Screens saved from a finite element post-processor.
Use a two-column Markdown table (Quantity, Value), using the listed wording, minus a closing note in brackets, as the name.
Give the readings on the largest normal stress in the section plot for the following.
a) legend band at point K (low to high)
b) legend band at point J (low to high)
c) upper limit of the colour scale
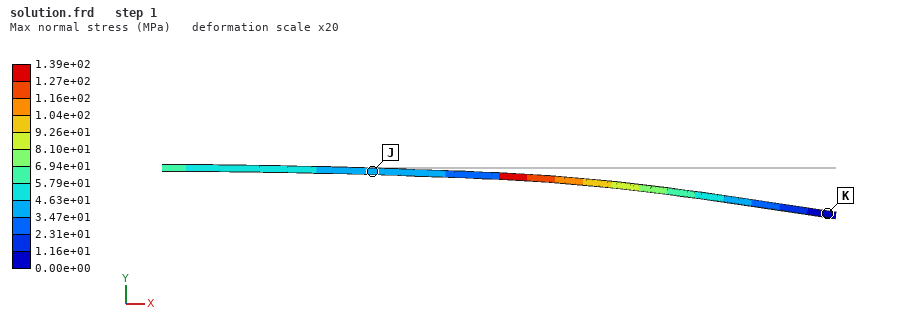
| Quantity | Value |
|---|---|
| legend band at point K | 0.00e+00 to 1.16e+01 MPa |
| legend band at point J | 3.47e+01 to 4.63e+01 MPa |
| upper limit of the colour scale | 1.39e+02 MPa |
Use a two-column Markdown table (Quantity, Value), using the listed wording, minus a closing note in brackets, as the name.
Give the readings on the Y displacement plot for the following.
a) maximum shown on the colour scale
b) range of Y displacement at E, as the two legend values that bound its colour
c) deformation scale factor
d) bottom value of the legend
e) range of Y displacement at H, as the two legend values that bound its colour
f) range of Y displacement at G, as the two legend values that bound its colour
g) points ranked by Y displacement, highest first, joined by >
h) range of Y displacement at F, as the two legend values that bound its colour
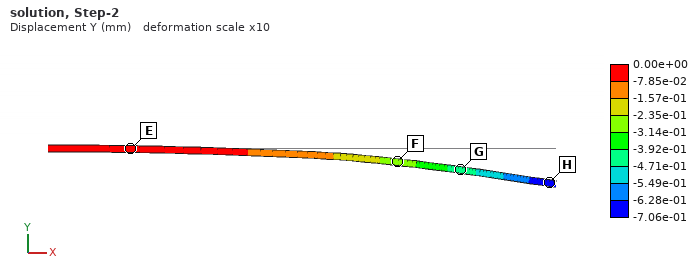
| Quantity | Value |
|---|---|
| maximum shown on the colour scale | 0.00e+00 mm |
| range of Y displacement at E, as the two legend values that bound its colour | -7.85e-02 to 0.00e+00 mm |
| deformation scale factor | 10 |
| bottom value of the legend | -7.06e-01 mm |
| range of Y displacement at H, as the two legend values that bound its colour | -7.06e-01 to -6.28e-01 mm |
| range of Y displacement at G, as the two legend values that bound its colour | -4.71e-01 to -3.92e-01 mm |
| points ranked by Y displacement, highest first, joined by > | E > F > G > H |
| range of Y displacement at F, as the two legend values that bound its colour | -3.14e-01 to -2.35e-01 mm |
